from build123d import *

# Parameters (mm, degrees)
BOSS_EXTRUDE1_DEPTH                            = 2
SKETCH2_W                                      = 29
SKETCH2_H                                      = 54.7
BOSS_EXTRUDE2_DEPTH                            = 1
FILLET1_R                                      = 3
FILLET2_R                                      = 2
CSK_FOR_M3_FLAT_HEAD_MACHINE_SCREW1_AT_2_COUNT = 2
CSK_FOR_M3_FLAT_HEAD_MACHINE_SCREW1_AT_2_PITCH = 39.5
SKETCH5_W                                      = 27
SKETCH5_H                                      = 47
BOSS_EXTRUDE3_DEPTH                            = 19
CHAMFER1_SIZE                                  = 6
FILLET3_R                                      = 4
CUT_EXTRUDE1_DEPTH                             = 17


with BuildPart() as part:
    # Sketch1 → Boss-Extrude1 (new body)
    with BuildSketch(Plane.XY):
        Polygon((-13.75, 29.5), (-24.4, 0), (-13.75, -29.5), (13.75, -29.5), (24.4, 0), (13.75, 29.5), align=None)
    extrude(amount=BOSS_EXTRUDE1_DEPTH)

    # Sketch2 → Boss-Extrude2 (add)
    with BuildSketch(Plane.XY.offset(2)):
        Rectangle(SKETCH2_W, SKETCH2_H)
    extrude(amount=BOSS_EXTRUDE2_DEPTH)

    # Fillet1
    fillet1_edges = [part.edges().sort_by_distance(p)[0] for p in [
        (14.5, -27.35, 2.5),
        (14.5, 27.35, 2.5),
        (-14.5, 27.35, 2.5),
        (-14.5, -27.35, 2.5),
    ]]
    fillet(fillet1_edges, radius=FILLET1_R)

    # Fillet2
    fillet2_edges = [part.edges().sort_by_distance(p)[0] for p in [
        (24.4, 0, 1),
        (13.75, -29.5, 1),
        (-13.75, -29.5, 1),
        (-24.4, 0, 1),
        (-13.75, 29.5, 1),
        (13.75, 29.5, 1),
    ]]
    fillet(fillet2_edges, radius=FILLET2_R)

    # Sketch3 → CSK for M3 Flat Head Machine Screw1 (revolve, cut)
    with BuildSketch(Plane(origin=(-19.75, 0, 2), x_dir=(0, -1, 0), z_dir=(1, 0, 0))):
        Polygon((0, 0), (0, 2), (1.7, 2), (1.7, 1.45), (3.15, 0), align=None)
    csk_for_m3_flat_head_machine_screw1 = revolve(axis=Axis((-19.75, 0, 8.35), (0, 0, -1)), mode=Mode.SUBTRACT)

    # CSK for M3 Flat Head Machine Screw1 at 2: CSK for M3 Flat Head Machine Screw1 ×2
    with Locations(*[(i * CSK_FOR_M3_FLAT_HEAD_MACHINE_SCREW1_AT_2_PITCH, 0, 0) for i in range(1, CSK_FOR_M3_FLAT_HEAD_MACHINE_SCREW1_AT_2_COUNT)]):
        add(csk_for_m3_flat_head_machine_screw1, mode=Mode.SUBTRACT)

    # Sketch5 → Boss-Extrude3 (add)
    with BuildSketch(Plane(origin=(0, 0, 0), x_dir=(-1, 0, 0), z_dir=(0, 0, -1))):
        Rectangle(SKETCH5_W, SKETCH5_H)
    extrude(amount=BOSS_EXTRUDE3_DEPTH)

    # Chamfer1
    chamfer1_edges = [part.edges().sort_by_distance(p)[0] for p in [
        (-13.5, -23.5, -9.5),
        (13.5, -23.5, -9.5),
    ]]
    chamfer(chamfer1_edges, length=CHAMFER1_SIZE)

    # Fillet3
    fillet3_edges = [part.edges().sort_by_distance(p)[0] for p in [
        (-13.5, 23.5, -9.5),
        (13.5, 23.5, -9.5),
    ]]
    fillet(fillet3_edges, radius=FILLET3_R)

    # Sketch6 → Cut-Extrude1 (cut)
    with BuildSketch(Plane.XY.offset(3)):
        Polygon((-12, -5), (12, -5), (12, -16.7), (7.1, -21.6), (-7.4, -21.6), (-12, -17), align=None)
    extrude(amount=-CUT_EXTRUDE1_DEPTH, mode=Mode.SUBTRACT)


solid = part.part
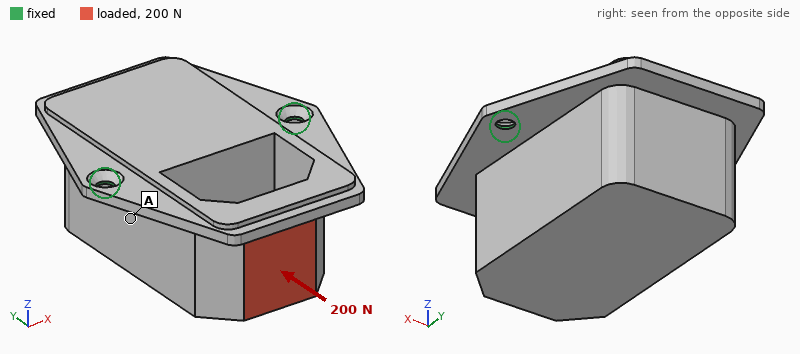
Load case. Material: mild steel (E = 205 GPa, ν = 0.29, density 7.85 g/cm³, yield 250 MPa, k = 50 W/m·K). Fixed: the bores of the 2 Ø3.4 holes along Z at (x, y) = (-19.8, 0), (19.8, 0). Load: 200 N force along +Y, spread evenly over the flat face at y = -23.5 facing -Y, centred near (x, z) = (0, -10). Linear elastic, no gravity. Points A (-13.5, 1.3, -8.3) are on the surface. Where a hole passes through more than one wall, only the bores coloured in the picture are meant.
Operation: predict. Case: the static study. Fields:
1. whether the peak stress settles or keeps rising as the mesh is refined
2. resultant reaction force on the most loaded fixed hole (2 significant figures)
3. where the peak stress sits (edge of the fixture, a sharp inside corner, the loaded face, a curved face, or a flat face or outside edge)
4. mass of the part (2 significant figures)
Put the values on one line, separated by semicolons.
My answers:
keeps rising; 100 N; edge of the fixture; 180 g
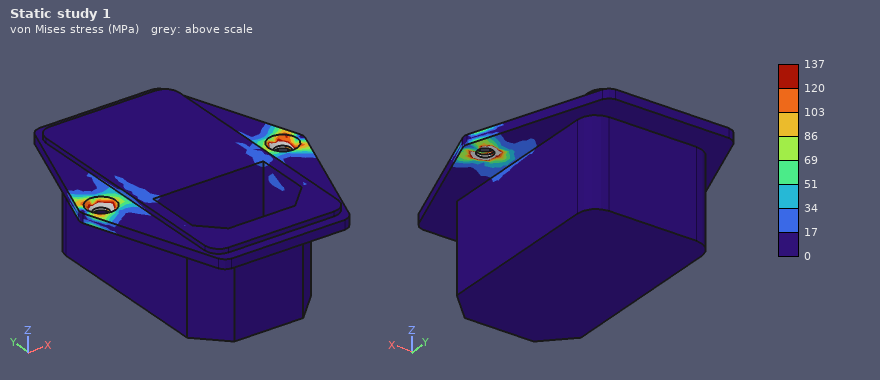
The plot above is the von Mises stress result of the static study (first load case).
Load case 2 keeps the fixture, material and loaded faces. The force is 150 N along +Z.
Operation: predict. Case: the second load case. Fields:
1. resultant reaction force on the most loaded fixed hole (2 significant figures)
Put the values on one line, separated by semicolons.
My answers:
83 N
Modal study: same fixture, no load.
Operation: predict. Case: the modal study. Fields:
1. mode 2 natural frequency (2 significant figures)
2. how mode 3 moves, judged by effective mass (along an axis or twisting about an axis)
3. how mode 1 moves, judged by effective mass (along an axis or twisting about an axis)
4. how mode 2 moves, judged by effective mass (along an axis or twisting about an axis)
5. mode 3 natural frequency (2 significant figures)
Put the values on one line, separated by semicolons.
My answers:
3500 Hz; along X; along Y; along Z; 3900 Hz
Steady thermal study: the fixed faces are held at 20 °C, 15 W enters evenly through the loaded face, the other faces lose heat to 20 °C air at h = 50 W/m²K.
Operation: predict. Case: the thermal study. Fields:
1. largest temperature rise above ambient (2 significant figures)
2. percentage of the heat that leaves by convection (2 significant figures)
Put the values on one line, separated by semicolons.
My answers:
52 K; 62 %
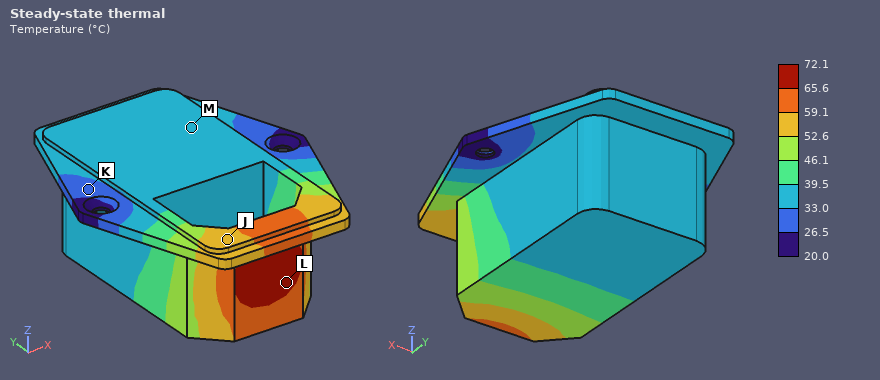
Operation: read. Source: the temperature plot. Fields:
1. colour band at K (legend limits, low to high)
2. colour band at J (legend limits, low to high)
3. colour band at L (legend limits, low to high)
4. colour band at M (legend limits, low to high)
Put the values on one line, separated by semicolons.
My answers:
26.5 to 33.0 °C; 52.6 to 59.1 °C; 65.6 to 72.1 °C; 33.0 to 39.5 °C
